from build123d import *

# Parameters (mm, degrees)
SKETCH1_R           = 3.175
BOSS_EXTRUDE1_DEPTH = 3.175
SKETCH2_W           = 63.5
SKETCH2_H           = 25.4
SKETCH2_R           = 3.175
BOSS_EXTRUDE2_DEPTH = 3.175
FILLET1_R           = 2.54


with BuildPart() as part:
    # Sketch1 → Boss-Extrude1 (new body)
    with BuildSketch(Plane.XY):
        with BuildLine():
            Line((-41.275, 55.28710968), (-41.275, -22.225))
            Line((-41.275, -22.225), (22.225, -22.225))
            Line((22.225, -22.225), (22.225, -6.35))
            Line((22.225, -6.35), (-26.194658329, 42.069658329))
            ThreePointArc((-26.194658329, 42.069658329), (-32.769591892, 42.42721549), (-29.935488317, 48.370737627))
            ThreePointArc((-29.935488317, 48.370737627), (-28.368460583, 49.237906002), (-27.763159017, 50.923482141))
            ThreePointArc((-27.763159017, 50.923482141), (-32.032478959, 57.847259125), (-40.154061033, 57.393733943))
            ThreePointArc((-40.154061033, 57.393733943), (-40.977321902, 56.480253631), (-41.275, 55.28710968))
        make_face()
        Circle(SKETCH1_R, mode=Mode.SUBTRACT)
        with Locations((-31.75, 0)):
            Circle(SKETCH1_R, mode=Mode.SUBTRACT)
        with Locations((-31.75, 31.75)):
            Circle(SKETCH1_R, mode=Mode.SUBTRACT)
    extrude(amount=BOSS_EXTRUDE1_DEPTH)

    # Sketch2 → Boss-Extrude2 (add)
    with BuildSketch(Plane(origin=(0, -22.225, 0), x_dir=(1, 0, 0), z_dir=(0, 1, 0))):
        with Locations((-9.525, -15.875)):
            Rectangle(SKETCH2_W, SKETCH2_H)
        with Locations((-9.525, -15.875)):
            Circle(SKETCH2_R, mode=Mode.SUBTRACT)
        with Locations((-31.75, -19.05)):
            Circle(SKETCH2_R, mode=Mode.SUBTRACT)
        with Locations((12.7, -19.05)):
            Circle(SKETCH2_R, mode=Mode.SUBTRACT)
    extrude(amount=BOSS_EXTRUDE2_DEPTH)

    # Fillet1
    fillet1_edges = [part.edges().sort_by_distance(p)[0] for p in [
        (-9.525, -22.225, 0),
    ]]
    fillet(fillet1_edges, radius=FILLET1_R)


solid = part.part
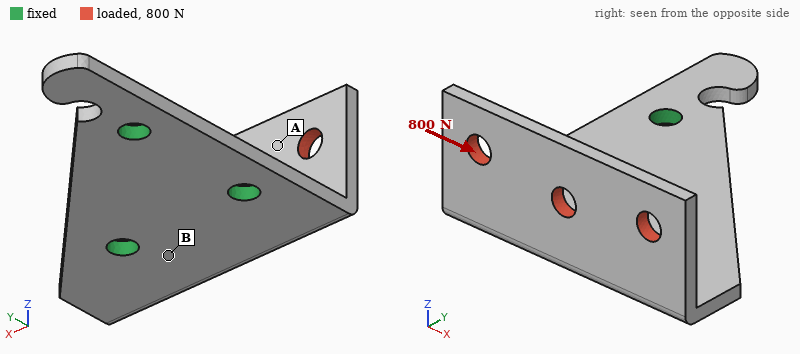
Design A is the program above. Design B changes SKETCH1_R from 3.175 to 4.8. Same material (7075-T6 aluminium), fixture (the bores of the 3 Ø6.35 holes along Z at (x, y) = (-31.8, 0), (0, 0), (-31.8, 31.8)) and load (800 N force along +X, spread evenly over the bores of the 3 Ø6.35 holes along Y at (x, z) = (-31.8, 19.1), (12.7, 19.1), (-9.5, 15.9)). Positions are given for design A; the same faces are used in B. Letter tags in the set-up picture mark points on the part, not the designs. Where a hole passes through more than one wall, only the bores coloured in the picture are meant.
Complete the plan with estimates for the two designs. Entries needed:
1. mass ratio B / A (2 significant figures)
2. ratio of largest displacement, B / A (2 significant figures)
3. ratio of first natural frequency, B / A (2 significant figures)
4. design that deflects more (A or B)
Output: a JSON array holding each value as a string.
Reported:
["0.97", "0.81", "1.1", "A"]
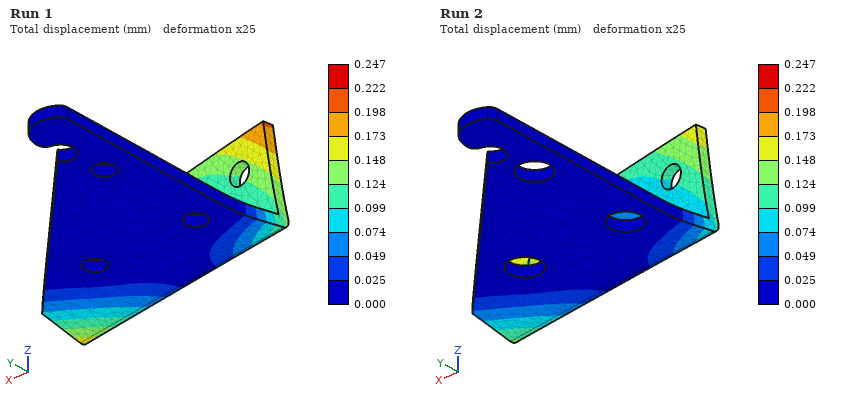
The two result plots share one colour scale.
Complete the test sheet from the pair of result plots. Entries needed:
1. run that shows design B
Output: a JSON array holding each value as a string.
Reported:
["Run 2"]
